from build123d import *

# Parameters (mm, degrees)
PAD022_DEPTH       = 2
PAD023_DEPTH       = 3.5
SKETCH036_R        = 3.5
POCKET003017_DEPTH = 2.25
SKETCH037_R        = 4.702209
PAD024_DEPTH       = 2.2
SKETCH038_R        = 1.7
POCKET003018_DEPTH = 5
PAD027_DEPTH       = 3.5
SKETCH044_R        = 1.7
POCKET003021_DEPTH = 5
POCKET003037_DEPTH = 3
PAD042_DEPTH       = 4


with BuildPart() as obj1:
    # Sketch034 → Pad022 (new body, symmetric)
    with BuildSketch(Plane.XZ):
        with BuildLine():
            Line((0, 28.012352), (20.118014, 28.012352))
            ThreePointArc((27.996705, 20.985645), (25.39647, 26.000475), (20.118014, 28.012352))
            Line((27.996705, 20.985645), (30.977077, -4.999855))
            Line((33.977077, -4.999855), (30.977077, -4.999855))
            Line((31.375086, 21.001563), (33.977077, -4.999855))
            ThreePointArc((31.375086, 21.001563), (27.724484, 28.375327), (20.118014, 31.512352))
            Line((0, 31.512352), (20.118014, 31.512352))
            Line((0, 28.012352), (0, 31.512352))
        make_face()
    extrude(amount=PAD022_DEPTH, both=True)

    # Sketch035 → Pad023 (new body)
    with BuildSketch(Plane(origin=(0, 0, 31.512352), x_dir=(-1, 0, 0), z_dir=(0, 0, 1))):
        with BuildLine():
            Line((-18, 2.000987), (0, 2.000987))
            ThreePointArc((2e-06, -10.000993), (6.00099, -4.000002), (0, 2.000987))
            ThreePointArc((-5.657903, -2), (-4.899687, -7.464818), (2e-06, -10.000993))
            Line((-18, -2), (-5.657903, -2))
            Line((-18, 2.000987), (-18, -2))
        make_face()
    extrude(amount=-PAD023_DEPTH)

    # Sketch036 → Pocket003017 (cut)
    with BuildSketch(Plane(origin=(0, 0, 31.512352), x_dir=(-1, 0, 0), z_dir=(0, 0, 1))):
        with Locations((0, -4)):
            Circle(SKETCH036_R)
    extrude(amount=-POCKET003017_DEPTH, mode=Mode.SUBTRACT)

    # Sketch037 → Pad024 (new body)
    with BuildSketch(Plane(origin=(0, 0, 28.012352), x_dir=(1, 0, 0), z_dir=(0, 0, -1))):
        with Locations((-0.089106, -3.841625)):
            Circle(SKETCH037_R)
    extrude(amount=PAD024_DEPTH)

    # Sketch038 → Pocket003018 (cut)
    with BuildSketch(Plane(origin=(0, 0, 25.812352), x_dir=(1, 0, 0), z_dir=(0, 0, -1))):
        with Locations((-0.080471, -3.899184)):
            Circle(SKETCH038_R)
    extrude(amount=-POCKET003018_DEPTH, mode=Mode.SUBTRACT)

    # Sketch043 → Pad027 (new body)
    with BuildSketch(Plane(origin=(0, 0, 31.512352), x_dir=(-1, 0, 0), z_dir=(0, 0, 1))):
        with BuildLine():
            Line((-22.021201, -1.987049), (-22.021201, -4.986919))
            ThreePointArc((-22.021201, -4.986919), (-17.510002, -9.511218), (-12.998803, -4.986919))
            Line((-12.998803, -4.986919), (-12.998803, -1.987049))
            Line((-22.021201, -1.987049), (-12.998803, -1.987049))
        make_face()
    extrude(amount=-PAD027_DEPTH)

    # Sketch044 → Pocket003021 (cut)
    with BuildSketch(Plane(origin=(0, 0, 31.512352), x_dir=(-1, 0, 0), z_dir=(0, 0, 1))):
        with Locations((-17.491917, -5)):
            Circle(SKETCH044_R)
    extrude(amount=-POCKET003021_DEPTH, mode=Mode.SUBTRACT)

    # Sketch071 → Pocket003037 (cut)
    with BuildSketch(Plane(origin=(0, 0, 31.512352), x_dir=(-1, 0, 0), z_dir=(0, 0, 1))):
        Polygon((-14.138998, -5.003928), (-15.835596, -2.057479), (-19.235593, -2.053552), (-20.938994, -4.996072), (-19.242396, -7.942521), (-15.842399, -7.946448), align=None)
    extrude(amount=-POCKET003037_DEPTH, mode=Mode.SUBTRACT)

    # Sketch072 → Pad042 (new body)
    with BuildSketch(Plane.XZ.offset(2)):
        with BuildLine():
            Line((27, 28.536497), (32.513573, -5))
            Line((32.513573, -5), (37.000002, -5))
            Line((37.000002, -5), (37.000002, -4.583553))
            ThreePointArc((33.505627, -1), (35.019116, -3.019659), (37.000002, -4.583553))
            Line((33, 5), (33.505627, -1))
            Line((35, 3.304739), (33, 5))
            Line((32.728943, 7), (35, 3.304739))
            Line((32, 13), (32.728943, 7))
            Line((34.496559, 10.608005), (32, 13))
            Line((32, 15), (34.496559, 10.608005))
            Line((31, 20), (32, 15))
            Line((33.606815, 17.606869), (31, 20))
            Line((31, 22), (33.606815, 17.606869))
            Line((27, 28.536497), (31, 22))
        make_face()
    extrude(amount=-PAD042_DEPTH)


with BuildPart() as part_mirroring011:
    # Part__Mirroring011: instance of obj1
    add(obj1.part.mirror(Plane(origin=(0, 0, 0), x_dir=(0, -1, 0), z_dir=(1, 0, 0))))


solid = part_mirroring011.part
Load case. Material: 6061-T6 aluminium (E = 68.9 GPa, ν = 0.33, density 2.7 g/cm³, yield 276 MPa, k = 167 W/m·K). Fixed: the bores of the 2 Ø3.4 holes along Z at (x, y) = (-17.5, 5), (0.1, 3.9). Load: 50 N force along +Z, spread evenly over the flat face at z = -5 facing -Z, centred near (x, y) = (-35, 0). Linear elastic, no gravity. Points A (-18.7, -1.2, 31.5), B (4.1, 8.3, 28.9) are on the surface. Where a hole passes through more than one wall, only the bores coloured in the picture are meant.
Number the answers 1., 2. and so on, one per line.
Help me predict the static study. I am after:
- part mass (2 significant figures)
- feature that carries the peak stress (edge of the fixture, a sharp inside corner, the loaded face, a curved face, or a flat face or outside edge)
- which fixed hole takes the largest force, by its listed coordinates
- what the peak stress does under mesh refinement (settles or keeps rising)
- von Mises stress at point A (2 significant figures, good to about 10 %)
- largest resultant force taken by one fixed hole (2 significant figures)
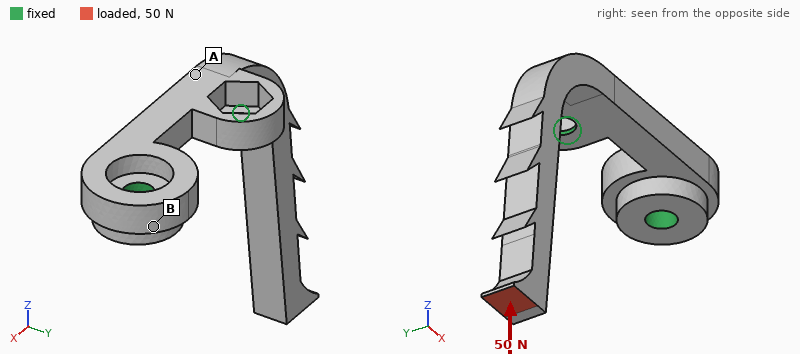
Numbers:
1. 3.6 g
2. edge of the fixture
3. (-17.5, 5)
4. keeps rising
5. 71 MPa
6. 110 N
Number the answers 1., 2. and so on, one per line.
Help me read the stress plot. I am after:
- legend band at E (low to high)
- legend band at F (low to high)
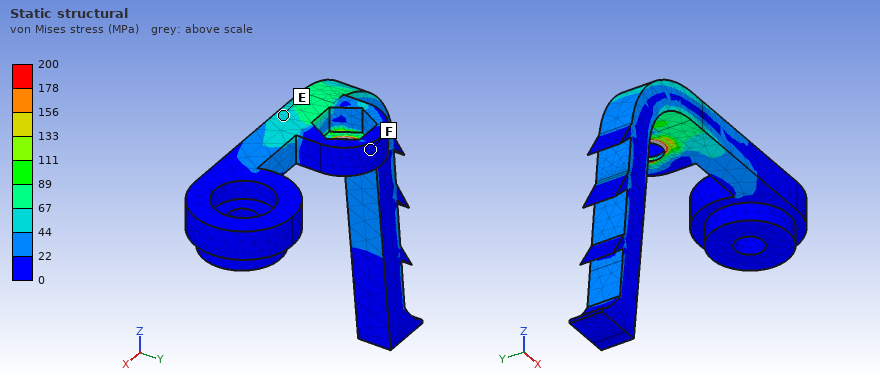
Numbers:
1. 44 to 67 MPa
2. 0 to 22 MPa
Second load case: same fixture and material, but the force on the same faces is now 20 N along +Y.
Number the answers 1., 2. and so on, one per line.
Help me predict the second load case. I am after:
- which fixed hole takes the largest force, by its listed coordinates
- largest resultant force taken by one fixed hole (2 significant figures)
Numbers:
1. (-17.5, 5)
2. 59 N
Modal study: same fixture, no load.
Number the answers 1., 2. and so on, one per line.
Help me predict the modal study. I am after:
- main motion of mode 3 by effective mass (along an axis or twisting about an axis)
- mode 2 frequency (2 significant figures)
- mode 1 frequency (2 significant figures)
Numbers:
1. along Z
2. 1500 Hz
3. 1300 Hz
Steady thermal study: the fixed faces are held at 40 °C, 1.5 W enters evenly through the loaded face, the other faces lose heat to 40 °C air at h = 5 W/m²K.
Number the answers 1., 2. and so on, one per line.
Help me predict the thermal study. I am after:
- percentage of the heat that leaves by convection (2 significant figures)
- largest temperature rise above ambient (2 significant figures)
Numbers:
1. 4.0 %
2. 31 K
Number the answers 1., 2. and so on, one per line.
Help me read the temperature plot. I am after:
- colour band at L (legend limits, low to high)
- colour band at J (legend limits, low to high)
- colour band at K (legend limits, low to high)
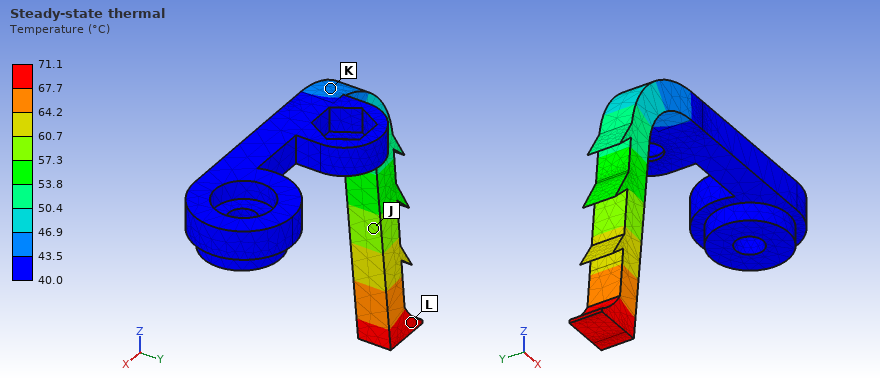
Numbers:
1. 67.7 to 71.1 °C
2. 57.3 to 60.7 °C
3. 43.5 to 46.9 °C
